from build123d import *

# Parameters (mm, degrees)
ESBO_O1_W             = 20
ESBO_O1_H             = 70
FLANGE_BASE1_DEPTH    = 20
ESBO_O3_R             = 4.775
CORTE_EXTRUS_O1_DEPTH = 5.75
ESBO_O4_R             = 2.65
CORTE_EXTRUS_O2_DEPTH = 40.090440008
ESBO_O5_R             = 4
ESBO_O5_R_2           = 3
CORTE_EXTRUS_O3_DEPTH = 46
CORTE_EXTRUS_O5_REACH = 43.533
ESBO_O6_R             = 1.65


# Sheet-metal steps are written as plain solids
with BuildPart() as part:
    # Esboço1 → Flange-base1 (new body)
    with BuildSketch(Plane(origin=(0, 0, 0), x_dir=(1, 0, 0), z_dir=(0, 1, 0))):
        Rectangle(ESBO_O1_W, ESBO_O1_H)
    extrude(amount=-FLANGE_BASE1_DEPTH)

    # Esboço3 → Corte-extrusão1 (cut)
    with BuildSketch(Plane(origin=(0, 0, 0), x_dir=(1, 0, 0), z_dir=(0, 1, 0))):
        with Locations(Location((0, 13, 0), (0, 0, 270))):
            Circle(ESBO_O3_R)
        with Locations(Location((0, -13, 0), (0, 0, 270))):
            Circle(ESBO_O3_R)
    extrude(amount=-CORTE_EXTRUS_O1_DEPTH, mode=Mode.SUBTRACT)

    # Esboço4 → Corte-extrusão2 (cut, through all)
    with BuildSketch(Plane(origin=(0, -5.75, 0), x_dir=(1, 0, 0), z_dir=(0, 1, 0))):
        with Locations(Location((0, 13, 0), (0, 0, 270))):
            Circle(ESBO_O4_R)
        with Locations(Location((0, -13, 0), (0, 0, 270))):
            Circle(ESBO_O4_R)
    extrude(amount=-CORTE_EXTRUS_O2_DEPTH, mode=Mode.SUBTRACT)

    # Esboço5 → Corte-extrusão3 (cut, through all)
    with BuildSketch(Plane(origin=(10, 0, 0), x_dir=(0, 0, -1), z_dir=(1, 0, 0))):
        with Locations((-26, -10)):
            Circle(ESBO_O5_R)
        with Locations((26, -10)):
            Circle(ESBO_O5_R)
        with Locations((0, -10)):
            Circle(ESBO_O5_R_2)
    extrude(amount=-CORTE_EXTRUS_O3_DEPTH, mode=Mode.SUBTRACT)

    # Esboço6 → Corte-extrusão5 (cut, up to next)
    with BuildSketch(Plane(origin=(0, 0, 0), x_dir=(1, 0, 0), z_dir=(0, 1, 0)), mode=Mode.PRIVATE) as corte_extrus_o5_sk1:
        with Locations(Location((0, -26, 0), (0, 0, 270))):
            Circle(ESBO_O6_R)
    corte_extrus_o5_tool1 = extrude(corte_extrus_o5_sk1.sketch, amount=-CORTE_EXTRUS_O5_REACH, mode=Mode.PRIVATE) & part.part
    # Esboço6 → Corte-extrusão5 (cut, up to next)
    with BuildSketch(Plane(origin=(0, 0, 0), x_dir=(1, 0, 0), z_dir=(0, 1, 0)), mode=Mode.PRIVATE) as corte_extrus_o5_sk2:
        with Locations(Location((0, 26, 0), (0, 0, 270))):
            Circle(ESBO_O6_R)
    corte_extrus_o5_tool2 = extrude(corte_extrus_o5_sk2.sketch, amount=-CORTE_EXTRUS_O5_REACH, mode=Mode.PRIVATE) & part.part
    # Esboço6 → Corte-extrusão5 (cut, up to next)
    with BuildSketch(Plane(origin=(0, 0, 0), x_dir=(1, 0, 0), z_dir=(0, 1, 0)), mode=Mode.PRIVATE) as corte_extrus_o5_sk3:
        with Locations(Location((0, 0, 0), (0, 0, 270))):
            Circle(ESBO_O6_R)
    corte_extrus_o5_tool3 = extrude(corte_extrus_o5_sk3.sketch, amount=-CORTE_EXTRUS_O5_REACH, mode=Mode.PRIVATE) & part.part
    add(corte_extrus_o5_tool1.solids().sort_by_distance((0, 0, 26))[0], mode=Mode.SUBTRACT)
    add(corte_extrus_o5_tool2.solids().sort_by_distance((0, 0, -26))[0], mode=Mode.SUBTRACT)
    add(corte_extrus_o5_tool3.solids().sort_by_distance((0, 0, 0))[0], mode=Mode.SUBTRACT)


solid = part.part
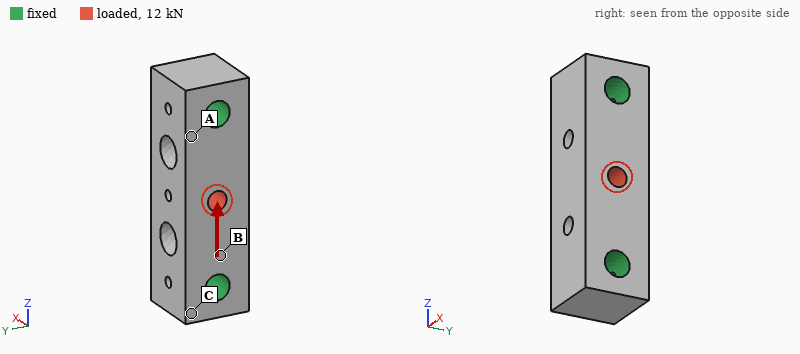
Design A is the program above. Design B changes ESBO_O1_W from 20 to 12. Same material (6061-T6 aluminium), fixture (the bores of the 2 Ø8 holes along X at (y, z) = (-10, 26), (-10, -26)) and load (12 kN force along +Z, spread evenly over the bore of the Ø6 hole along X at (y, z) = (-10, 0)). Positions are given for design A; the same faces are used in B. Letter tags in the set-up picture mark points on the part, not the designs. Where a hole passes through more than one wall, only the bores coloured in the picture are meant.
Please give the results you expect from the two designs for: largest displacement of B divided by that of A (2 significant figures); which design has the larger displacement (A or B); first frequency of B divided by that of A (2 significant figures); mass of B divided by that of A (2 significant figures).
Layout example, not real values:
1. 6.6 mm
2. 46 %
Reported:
1. 2.0
2. B
3. 0.74
4. 0.57
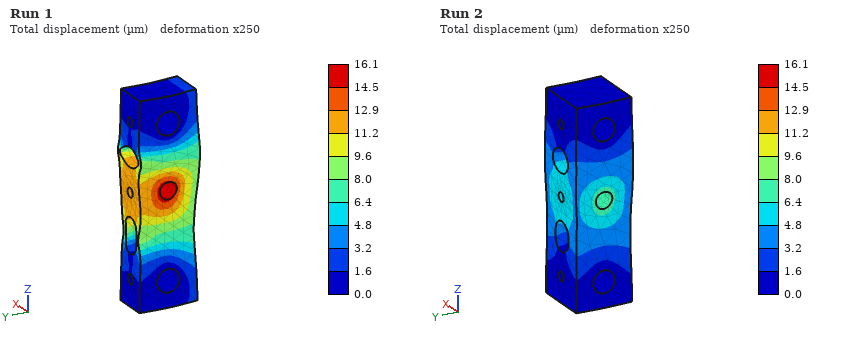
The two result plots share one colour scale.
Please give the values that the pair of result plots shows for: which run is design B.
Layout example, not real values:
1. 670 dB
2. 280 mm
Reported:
1. Run 1
